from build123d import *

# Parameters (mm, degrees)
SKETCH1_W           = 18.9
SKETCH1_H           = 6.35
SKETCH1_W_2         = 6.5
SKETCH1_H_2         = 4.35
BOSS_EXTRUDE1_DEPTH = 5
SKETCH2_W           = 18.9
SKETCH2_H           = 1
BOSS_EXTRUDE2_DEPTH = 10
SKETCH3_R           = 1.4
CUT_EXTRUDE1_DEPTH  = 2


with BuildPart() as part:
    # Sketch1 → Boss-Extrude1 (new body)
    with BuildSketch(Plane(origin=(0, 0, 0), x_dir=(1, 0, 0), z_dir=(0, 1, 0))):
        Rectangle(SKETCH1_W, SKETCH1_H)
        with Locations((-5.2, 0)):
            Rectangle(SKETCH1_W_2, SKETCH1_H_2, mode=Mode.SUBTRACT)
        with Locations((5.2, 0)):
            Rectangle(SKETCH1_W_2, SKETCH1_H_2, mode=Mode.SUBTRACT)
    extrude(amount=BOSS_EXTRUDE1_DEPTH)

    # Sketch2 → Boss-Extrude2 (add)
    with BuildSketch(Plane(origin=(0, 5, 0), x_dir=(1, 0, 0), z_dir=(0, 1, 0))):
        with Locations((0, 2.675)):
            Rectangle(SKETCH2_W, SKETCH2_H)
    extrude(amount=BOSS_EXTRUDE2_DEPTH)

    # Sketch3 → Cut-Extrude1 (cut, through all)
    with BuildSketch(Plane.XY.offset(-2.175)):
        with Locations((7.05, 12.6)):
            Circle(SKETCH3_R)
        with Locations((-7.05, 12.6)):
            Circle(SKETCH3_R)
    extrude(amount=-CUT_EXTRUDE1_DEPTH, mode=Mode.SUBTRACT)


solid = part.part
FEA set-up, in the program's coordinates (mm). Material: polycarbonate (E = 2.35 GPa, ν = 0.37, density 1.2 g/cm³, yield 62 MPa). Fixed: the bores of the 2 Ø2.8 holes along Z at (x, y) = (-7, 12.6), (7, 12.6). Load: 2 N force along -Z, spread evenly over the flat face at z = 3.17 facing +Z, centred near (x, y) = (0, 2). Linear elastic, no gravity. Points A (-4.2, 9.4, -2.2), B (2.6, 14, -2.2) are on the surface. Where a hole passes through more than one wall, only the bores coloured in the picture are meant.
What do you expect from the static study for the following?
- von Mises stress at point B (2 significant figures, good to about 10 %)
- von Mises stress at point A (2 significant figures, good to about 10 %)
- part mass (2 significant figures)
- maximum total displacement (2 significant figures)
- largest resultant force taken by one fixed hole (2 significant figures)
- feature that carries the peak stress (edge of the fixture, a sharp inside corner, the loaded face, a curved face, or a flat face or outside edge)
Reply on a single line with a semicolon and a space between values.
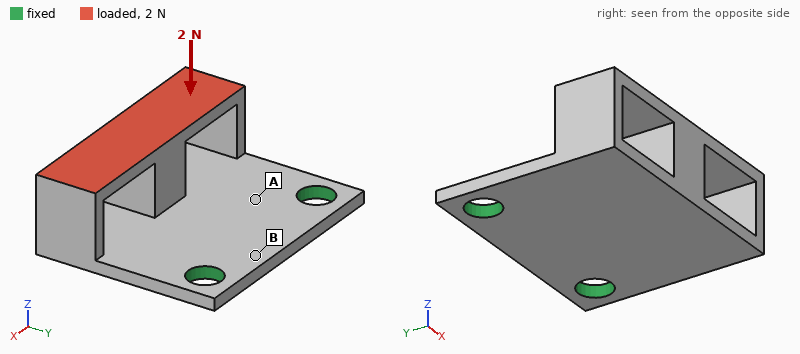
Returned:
1.4 MPa; 3.7 MPa; 0.59 g; 0.25 mm; 1.0 N; a flat face or outside edge
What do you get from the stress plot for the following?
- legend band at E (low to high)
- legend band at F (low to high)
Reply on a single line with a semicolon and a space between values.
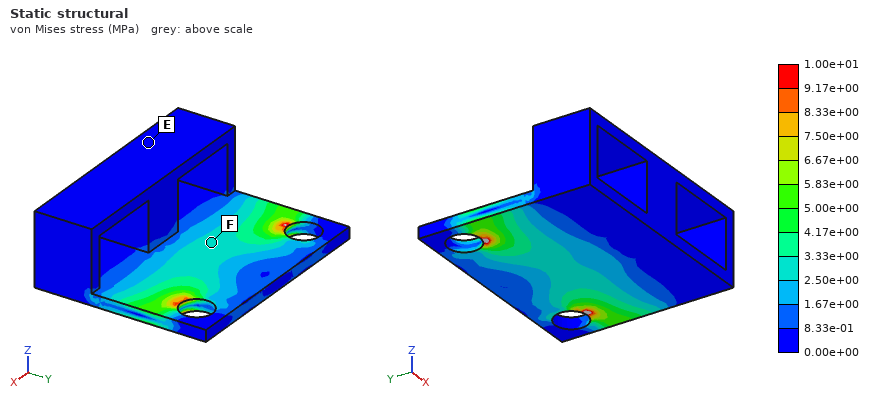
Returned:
0.00e+00 to 8.33e-01 MPa; 2.50e+00 to 3.33e+00 MPa
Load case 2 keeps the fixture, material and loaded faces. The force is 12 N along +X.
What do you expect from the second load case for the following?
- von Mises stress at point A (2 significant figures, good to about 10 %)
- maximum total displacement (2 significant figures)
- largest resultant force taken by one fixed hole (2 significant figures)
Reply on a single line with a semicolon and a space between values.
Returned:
6.6 MPa; 0.29 mm; 11 N
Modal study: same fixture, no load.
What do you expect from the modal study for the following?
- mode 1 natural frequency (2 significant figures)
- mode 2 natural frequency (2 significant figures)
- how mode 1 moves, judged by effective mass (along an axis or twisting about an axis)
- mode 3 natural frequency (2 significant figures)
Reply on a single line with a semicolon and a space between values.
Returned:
810 Hz; 2100 Hz; along Z; 3800 Hz
